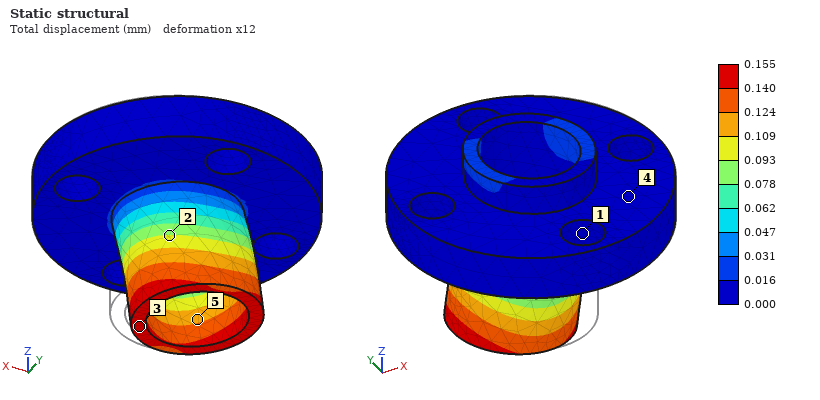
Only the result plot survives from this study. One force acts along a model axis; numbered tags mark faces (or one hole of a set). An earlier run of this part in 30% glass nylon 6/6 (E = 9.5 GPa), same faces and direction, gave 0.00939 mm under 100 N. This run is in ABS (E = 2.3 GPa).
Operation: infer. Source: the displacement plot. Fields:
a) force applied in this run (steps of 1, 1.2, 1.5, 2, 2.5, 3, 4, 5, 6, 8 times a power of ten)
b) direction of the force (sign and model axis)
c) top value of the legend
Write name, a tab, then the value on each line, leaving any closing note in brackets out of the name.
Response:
force applied in this run	400 N
direction of the force	-X
top value of the legend	0.155 mm
